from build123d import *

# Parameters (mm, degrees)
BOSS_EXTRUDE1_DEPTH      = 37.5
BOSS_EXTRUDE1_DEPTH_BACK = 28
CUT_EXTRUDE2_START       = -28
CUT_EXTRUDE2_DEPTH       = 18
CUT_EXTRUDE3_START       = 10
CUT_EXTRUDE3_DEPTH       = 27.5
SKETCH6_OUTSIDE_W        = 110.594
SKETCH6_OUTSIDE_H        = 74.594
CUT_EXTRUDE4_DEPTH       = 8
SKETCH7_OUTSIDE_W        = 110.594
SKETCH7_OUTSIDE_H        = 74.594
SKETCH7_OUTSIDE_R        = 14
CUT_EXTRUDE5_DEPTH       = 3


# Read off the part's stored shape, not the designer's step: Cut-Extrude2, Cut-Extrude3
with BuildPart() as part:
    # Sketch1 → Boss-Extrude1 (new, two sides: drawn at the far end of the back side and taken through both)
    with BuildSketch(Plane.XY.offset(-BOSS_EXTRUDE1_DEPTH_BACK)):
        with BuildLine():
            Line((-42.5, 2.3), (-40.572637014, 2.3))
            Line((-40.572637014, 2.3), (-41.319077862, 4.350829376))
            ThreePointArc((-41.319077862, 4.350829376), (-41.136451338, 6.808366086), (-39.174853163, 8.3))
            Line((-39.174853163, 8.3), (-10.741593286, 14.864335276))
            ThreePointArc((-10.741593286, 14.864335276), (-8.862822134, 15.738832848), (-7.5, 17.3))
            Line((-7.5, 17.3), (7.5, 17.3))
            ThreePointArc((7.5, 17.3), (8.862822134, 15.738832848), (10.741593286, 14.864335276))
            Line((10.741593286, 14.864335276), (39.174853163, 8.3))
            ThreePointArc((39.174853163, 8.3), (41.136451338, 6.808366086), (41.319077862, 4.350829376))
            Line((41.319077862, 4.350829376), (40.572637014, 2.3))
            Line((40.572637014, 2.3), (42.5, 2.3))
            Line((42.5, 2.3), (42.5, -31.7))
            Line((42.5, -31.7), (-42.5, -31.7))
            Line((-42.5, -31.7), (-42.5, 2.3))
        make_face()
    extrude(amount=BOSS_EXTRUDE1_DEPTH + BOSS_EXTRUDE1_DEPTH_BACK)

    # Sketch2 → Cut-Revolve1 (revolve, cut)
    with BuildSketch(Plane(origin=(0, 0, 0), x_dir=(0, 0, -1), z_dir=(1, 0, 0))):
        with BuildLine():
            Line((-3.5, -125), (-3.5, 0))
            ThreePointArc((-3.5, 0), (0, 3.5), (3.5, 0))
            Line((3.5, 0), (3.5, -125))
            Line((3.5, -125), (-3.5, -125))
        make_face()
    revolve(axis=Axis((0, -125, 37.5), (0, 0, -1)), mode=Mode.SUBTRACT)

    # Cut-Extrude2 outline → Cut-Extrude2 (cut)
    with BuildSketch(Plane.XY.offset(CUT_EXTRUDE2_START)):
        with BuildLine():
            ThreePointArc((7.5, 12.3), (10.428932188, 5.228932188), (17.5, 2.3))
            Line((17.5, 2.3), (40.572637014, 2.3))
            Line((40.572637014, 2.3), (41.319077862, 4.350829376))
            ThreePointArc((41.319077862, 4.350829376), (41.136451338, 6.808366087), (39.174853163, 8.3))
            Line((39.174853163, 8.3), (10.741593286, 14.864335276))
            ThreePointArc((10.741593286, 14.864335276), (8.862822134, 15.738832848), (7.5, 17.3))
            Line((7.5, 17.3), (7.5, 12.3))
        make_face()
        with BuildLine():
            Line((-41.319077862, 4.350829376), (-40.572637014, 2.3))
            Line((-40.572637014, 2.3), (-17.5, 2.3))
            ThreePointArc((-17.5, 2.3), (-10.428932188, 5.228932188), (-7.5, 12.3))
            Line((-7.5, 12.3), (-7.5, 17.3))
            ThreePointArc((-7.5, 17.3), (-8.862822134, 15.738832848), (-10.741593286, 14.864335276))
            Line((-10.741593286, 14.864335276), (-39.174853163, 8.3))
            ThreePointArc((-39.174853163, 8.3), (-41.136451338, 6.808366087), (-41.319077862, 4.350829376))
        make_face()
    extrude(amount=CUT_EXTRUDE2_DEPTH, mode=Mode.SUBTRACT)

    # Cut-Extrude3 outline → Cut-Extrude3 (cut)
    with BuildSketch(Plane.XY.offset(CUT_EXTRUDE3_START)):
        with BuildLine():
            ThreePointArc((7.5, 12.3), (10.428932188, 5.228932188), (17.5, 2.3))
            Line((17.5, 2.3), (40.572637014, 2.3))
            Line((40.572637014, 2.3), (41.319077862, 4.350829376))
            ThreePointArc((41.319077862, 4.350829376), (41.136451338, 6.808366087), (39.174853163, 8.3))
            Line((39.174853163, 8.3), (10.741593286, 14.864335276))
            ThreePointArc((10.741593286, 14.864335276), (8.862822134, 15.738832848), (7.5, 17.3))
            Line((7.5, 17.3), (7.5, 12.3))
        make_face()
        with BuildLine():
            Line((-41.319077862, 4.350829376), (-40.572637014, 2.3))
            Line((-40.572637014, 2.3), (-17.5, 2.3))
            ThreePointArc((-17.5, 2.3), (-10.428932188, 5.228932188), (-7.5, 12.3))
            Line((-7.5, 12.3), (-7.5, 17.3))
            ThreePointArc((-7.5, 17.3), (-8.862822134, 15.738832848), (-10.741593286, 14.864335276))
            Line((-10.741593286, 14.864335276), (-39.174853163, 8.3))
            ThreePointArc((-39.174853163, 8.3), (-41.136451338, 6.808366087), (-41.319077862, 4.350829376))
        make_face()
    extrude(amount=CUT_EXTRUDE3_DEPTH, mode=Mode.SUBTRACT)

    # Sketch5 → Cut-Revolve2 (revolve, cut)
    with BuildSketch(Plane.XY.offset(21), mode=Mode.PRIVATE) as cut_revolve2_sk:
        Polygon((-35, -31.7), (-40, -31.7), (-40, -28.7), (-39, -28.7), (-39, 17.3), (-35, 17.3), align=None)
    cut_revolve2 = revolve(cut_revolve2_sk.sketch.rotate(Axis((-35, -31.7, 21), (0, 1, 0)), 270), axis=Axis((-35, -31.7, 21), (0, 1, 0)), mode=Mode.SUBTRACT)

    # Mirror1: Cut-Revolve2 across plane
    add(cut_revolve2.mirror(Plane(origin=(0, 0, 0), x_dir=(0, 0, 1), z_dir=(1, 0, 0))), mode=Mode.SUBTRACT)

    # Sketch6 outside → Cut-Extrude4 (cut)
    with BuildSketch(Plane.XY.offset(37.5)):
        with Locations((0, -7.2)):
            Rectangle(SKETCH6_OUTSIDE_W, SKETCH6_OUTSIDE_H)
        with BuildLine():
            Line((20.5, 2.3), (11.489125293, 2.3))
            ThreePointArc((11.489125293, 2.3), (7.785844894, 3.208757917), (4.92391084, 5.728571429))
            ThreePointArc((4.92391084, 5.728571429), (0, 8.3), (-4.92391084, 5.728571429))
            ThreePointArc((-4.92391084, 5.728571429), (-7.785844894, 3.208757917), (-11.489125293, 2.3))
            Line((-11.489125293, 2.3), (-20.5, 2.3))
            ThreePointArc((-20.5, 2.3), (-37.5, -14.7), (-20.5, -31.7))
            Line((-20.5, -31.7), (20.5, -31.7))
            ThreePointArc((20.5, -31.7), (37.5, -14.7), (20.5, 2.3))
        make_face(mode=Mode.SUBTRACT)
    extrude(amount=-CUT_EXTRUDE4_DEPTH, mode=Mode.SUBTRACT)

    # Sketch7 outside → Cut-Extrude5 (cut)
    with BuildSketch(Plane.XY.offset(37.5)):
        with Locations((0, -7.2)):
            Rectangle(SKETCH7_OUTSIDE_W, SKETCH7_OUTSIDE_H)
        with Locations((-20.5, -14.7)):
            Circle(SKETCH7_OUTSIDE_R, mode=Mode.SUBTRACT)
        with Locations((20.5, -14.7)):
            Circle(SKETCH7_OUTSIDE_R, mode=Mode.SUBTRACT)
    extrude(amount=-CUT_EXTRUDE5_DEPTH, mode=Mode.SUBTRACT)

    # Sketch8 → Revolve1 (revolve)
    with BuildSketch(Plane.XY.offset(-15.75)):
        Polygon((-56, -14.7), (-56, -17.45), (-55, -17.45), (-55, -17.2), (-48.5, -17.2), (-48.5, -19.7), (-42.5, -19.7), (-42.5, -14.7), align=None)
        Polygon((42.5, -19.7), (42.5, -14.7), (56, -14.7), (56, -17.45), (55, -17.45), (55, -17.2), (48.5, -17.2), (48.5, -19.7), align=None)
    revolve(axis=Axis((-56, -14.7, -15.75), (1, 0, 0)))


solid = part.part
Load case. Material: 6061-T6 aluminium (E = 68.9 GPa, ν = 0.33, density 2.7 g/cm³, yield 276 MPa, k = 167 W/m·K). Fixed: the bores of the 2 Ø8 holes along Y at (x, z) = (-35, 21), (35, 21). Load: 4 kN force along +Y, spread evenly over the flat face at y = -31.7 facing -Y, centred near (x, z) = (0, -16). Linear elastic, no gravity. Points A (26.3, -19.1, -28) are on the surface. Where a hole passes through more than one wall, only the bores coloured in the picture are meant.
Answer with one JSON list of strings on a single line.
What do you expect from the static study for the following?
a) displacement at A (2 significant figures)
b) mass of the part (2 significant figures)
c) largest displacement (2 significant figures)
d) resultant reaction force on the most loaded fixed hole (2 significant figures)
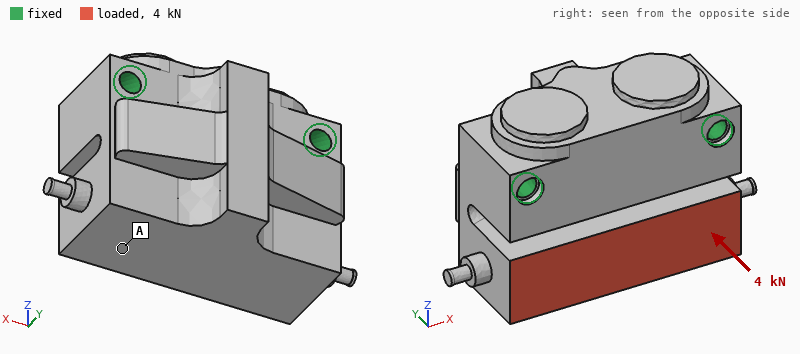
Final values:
["0.10 mm", "510 g", "0.12 mm", "2.0 kN"]
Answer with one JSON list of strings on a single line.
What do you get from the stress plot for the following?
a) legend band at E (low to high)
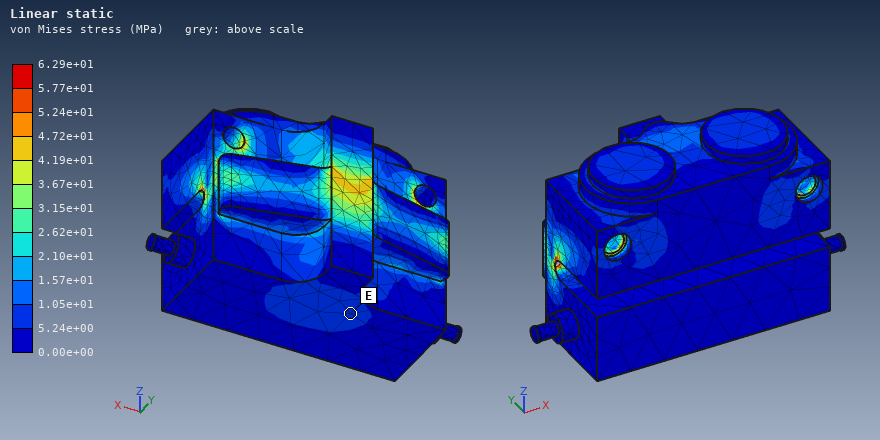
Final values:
["5.24e+00 to 1.05e+01 MPa"]
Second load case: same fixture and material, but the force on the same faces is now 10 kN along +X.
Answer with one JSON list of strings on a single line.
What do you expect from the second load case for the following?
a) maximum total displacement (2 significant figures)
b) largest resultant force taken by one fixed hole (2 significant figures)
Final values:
["0.13 mm", "7.6 kN"]
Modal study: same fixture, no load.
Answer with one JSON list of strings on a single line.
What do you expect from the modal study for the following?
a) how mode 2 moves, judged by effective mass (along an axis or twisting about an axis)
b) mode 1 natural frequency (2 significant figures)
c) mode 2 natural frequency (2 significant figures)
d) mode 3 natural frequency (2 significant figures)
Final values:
["along X", "2100 Hz", "4300 Hz", "5900 Hz"]
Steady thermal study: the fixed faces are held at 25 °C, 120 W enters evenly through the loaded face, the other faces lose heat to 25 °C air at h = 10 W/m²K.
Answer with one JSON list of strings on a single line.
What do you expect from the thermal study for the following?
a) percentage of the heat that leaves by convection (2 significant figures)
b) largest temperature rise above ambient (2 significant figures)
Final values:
["3.4 %", "37 K"]
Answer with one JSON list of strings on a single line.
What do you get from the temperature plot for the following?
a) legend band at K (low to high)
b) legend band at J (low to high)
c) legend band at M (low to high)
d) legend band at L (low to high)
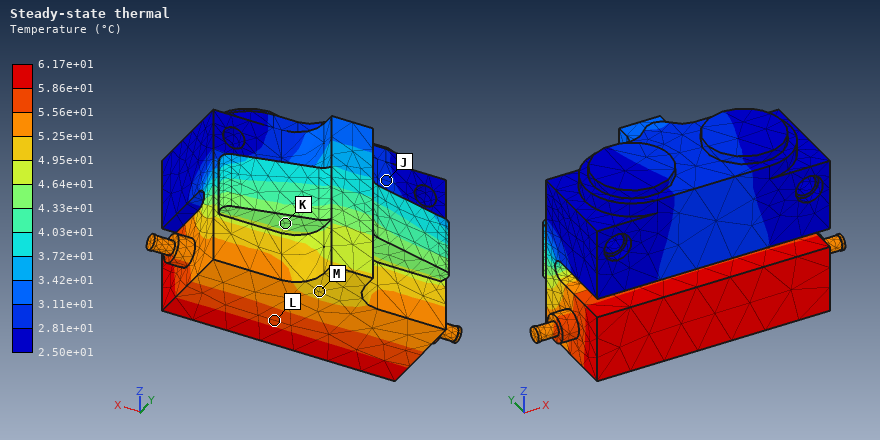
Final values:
["4.33e+01 to 4.64e+01 °C", "2.81e+01 to 3.11e+01 °C", "4.95e+01 to 5.25e+01 °C", "5.56e+01 to 5.86e+01 °C"]
